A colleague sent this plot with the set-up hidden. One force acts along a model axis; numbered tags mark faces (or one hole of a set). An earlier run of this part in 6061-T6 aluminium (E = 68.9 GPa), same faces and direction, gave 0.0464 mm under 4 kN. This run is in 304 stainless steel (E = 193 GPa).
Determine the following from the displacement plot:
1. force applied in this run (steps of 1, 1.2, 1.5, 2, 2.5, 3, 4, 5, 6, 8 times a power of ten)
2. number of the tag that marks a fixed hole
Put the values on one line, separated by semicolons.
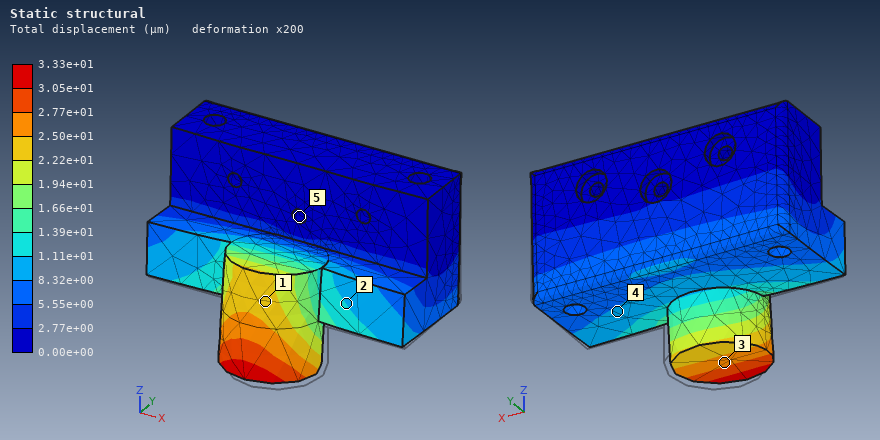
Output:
8 kN; 5
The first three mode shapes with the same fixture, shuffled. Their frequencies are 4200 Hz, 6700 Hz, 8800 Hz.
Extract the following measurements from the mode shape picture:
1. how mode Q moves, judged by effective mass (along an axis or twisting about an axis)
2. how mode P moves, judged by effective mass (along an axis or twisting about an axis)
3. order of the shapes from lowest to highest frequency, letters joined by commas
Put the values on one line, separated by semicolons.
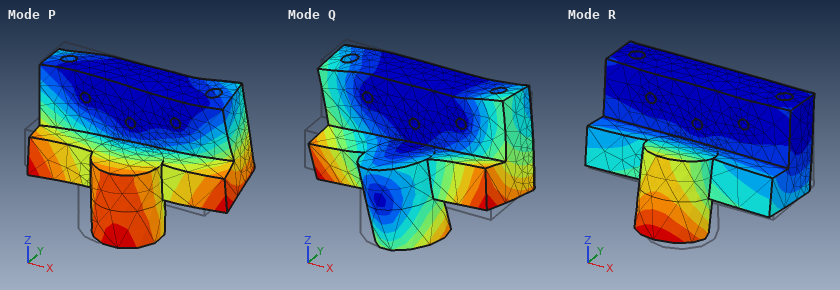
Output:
along X; along X; R, P, Q
